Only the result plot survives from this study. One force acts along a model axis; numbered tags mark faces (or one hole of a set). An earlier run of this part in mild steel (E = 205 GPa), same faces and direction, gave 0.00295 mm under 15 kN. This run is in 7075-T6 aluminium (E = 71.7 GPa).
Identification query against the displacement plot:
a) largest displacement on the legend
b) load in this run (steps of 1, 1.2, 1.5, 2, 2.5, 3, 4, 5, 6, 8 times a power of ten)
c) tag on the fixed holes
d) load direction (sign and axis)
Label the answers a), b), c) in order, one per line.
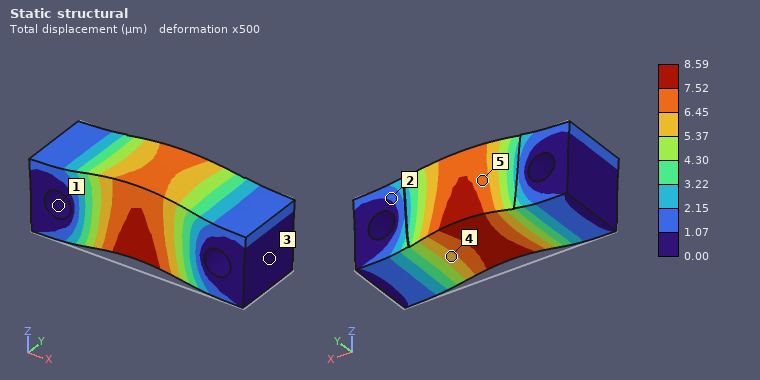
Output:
a) 8.59 µm
b) 15 kN
c) 1
d) +Z
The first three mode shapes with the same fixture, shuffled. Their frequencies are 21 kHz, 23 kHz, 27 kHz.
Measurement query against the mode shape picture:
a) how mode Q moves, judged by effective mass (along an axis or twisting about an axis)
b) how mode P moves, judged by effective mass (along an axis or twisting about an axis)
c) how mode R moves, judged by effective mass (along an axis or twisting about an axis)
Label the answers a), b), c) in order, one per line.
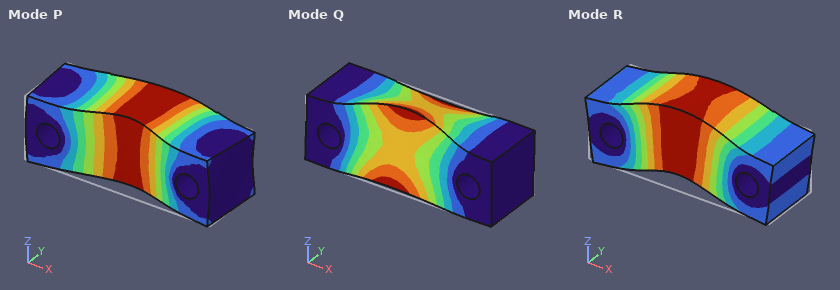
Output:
a) twisting about X
b) along Y
c) along Z
